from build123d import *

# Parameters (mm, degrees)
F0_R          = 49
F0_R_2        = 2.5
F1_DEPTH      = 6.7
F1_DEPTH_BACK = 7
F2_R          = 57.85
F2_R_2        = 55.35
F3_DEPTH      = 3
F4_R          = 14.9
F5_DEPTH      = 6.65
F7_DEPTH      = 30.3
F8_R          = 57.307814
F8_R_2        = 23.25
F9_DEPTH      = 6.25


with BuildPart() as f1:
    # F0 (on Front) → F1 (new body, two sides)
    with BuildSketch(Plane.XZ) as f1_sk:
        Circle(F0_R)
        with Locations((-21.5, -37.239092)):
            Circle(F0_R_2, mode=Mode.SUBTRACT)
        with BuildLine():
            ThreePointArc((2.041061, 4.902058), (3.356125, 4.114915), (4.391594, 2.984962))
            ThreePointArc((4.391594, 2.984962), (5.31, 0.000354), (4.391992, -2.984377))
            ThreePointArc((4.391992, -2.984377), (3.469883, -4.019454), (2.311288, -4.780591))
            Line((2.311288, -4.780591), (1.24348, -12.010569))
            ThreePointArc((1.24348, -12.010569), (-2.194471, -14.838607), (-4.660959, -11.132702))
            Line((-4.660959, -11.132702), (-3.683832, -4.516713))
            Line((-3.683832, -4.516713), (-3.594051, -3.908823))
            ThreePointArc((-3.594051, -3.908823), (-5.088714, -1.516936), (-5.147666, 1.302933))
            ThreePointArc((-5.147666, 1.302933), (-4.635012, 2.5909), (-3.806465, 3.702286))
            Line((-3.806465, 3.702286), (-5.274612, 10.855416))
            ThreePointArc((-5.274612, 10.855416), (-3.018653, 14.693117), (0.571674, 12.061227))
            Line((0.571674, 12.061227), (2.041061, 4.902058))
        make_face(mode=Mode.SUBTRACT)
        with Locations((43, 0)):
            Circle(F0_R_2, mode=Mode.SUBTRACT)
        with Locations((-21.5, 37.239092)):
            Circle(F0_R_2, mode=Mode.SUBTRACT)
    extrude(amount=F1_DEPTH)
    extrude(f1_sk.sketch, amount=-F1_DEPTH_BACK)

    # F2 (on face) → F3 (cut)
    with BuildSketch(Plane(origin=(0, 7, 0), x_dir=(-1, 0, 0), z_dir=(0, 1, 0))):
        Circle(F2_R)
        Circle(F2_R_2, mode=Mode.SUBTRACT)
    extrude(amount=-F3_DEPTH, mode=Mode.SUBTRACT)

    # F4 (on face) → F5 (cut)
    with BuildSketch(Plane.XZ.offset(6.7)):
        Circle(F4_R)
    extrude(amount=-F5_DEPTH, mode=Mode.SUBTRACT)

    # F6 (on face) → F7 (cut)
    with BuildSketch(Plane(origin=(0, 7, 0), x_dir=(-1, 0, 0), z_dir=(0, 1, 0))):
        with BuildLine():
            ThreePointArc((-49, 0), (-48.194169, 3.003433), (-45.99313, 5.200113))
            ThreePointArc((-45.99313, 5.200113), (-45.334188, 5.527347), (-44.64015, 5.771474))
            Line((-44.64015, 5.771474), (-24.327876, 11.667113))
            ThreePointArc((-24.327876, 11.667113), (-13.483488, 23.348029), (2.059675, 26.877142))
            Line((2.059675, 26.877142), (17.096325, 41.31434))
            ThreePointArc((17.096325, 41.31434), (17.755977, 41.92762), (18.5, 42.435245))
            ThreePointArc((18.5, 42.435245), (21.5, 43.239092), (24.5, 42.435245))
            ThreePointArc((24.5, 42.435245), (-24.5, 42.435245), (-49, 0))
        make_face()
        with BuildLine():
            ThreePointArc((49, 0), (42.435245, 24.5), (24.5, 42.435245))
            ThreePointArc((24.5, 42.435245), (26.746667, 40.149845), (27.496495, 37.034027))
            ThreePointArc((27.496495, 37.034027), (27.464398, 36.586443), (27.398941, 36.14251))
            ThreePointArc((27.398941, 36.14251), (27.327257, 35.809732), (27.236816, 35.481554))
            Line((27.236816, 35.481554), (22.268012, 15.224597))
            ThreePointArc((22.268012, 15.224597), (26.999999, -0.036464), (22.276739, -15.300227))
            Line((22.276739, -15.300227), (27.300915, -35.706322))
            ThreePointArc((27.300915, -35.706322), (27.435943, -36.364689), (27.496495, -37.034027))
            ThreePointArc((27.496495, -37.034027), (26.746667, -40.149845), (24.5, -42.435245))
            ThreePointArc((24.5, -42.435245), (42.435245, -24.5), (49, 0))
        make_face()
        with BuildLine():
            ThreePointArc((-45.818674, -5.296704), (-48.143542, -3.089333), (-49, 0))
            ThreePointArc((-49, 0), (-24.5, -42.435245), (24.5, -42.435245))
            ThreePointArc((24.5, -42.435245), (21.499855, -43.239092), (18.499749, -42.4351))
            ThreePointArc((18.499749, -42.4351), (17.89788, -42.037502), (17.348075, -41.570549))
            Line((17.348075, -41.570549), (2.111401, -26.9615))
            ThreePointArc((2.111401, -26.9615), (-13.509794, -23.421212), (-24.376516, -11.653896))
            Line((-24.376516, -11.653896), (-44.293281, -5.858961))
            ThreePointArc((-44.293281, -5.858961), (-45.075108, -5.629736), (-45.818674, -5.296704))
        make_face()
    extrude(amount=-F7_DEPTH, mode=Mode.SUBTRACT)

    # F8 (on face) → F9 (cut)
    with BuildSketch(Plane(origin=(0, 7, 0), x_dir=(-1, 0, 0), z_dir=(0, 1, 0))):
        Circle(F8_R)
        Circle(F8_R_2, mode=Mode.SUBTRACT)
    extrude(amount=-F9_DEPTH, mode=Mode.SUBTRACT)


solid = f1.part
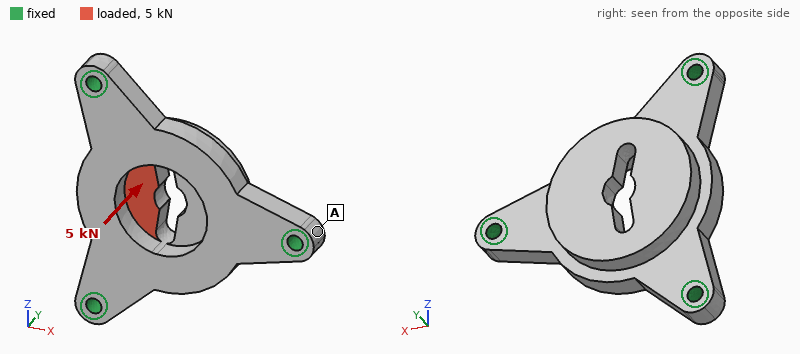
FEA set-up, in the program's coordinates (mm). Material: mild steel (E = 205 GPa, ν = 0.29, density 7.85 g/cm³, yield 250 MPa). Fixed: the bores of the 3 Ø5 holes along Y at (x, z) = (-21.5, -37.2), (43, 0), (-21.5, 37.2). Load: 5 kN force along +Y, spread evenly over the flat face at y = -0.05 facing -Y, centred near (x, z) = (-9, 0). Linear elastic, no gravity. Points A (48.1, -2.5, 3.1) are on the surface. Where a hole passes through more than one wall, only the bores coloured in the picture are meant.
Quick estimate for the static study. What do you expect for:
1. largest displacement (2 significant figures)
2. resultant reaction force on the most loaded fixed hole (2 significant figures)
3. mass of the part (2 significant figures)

40 µm
2.8 kN
230 g
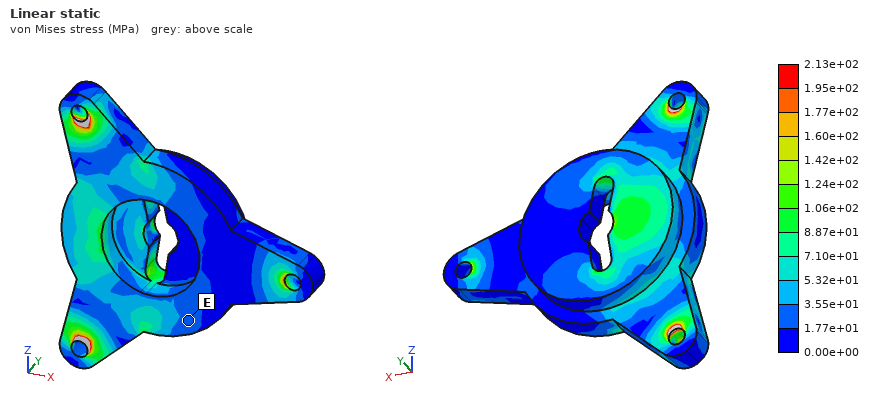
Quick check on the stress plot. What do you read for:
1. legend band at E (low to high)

1.77e+01 to 3.55e+01 MPa
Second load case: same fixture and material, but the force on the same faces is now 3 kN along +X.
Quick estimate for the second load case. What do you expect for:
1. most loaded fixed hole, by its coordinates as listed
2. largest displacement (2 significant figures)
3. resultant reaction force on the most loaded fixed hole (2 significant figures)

(43, 0)
8.1 µm
1.4 kN
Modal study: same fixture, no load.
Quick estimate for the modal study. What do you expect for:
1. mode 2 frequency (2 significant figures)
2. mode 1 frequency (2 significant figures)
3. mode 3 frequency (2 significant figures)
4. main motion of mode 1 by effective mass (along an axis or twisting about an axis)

8700 Hz
5800 Hz
8700 Hz
along Y
